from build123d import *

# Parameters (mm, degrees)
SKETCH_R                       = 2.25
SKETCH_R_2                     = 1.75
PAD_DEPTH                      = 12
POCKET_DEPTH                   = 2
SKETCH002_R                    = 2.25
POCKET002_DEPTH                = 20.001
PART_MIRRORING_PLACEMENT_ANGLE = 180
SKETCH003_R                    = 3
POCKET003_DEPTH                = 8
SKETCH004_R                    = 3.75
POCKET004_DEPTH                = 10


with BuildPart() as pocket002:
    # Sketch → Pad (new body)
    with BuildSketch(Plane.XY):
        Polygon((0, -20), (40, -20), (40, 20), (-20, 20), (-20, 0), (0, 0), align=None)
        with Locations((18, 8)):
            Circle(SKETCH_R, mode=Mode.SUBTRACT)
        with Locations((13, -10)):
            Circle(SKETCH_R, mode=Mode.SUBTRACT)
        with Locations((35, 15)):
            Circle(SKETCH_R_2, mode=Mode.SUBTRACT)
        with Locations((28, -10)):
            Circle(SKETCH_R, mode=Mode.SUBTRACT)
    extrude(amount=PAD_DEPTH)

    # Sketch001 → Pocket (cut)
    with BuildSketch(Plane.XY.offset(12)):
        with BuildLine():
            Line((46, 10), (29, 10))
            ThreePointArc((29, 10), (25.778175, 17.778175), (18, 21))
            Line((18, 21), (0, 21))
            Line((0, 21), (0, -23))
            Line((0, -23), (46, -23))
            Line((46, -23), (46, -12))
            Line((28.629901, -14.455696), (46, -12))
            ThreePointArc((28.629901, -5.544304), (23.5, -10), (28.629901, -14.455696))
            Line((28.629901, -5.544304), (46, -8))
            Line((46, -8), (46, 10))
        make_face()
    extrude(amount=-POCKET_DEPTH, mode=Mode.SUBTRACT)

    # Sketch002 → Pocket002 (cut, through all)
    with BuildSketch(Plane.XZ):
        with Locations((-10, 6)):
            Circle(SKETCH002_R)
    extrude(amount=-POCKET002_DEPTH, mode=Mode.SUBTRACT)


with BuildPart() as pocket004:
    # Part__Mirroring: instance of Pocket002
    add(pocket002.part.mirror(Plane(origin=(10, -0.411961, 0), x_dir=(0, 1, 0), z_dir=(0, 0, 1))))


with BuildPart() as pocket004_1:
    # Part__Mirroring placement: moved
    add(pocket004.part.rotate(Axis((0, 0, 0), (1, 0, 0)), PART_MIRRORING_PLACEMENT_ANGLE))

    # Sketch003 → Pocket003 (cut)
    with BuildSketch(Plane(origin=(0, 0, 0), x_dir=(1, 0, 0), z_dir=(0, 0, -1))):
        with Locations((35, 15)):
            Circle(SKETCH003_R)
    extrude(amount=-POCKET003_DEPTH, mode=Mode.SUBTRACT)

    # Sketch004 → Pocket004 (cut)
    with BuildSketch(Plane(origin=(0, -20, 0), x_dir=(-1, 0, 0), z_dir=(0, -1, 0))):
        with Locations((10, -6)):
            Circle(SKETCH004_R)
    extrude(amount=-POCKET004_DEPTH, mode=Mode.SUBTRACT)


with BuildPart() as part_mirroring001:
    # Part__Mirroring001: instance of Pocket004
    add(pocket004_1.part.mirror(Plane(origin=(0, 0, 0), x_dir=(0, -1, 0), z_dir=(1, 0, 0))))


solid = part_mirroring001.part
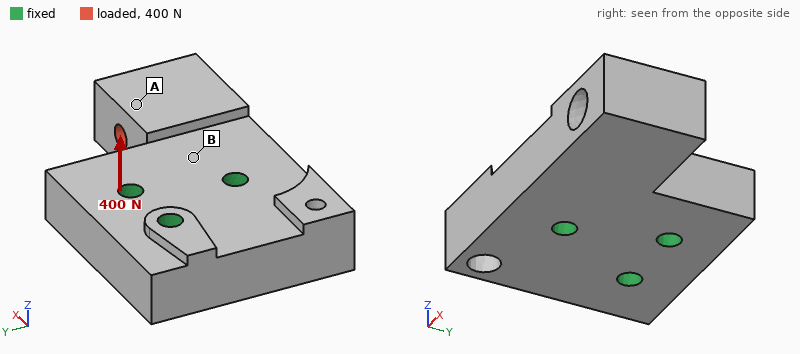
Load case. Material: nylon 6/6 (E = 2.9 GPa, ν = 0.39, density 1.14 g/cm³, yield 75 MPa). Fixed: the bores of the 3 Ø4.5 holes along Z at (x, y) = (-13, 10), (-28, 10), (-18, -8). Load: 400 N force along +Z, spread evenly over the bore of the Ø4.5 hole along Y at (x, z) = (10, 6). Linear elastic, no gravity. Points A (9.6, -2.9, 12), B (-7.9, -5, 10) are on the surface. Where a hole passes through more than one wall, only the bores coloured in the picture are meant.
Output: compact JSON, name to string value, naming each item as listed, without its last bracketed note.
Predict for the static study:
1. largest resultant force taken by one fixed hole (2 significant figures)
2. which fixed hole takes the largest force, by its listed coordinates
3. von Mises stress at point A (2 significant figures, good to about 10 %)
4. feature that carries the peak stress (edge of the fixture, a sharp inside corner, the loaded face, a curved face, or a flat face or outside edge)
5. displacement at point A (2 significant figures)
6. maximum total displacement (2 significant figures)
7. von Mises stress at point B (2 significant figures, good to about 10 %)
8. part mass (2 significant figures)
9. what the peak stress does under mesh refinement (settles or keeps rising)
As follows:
{"largest resultant force taken by one fixed hole": "290 N", "which fixed hole takes the largest force, by its listed coordinates": "(-13, 10)", "von Mises stress at point A": "3.2 MPa", "feature that carries the peak stress": "edge of the fixture", "displacement at point A": "0.48 mm", "maximum total displacement": "0.71 mm", "von Mises stress at point B": "16 MPa", "part mass": "23 g", "what the peak stress does under mesh refinement": "keeps rising"}
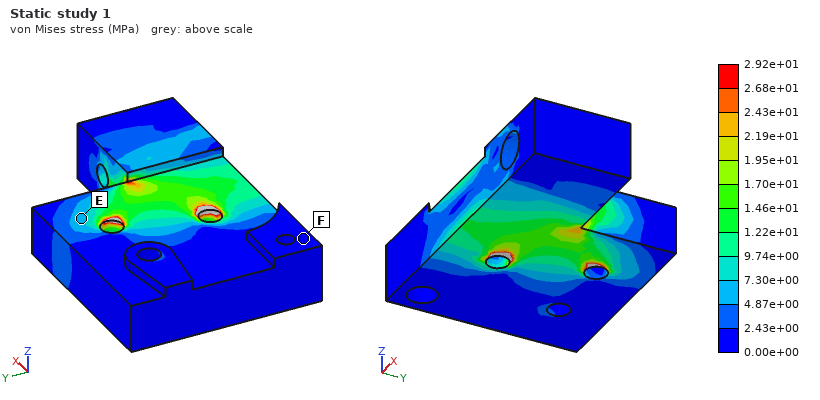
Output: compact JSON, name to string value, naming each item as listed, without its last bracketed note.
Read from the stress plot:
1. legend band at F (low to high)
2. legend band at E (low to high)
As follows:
{"legend band at F": "0.00e+00 to 2.43e+00 MPa", "legend band at E": "4.87e+00 to 7.30e+00 MPa"}
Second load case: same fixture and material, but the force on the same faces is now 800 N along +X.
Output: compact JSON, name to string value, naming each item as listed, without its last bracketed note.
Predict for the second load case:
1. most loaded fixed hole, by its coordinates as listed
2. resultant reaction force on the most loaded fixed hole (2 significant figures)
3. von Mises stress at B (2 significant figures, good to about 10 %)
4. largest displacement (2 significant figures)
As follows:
{"most loaded fixed hole, by its coordinates as listed": "(-18, -8)", "resultant reaction force on the most loaded fixed hole": "620 N", "von Mises stress at B": "7.0 MPa", "largest displacement": "0.11 mm"}
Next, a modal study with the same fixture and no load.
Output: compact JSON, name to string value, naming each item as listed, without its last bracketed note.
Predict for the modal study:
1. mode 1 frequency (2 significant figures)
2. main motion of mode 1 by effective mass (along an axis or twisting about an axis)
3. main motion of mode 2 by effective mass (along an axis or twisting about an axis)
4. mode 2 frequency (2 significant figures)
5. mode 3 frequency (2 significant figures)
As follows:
{"mode 1 frequency": "1900 Hz", "main motion of mode 1 by effective mass": "along Z", "main motion of mode 2 by effective mass": "along Y", "mode 2 frequency": "4000 Hz", "mode 3 frequency": "5600 Hz"}
